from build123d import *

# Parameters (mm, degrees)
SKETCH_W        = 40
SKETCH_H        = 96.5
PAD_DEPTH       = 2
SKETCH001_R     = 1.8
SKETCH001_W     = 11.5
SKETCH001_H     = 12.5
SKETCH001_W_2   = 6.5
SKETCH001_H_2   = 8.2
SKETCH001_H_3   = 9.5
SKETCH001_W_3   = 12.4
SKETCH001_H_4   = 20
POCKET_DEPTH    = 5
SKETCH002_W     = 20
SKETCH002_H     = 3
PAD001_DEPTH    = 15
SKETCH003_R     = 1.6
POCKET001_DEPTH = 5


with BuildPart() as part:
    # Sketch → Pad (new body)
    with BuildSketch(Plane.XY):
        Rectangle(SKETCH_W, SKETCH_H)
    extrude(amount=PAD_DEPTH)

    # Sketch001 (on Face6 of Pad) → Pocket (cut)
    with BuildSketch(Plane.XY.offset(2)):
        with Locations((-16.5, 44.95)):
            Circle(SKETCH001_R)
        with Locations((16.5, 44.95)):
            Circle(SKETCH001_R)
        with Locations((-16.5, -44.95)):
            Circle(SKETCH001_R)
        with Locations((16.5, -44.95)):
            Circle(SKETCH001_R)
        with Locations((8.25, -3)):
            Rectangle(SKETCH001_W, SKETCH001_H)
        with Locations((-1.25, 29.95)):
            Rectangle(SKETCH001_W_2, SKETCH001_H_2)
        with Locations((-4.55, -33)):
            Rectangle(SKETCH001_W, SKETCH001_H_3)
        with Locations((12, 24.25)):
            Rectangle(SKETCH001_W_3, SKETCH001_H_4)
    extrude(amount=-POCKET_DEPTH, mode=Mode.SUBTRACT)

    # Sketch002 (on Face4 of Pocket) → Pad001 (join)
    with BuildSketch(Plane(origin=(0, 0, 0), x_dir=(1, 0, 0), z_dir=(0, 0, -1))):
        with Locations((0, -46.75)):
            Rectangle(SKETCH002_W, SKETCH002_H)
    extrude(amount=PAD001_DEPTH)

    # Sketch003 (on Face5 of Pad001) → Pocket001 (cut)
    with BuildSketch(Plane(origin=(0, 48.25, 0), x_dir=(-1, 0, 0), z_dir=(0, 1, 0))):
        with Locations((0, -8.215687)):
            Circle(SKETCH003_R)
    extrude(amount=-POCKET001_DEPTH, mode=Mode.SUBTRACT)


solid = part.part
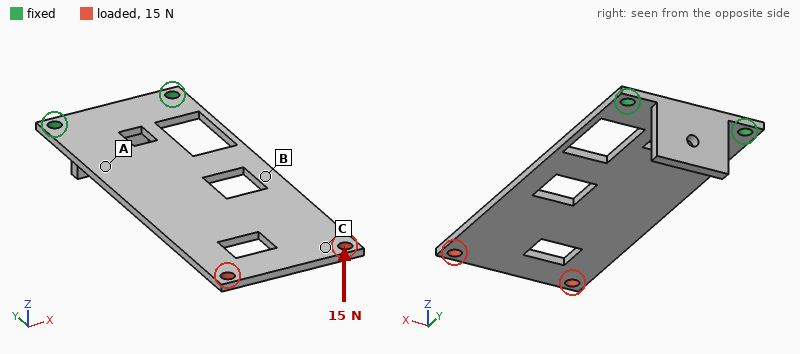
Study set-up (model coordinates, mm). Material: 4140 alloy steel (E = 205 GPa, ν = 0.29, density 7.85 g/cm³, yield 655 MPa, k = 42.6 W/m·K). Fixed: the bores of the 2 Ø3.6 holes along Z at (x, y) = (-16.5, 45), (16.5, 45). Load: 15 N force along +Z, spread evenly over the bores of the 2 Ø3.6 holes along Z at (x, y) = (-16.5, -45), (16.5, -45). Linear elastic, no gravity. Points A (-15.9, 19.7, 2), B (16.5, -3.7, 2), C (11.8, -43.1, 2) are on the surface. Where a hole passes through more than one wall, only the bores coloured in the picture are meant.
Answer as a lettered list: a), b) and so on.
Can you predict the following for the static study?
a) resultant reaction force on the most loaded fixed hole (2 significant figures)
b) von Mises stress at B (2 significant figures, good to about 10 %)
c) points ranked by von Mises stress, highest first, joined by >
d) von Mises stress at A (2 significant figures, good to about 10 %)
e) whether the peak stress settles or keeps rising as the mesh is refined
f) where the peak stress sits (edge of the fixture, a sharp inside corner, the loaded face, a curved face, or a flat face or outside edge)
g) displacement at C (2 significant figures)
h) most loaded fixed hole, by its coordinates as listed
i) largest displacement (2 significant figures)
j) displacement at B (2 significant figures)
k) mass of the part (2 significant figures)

a) 12 N
b) 33 MPa
c) A > B > C
d) 55 MPa
e) keeps rising
f) edge of the fixture
g) 0.99 mm
h) (-16.5, 45)
i) 1.1 mm
j) 0.38 mm
k) 58 g
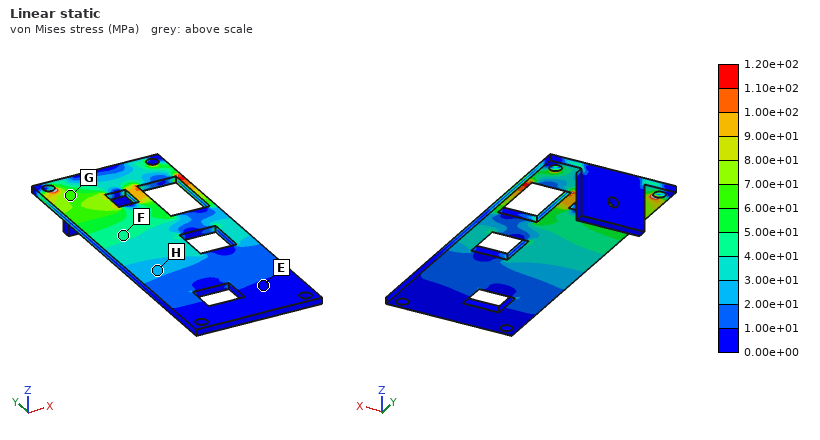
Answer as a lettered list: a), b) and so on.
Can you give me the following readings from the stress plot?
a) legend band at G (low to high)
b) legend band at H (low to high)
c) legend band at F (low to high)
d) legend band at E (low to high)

a) 6.00e+01 to 7.00e+01 MPa
b) 2.00e+01 to 3.00e+01 MPa
c) 4.00e+01 to 5.00e+01 MPa
d) 0.00e+00 to 1.00e+01 MPa
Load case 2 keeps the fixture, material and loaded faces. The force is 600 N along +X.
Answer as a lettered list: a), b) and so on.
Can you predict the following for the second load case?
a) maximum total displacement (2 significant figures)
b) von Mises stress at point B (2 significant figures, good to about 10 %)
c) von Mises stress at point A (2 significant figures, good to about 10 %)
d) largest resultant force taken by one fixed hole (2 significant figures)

a) 0.16 mm
b) 68 MPa
c) 65 MPa
d) 1.7 kN
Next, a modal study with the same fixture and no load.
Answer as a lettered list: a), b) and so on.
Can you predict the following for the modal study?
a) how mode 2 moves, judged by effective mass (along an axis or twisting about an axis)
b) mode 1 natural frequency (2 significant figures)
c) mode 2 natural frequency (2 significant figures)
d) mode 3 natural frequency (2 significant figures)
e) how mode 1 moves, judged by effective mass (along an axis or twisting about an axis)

a) twisting about Y
b) 160 Hz
c) 840 Hz
d) 1100 Hz
e) along Z
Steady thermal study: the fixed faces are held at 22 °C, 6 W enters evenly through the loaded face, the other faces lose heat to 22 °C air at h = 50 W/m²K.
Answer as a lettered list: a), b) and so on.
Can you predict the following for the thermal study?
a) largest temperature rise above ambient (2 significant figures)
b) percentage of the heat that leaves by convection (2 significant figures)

a) 68 K
b) 96 %
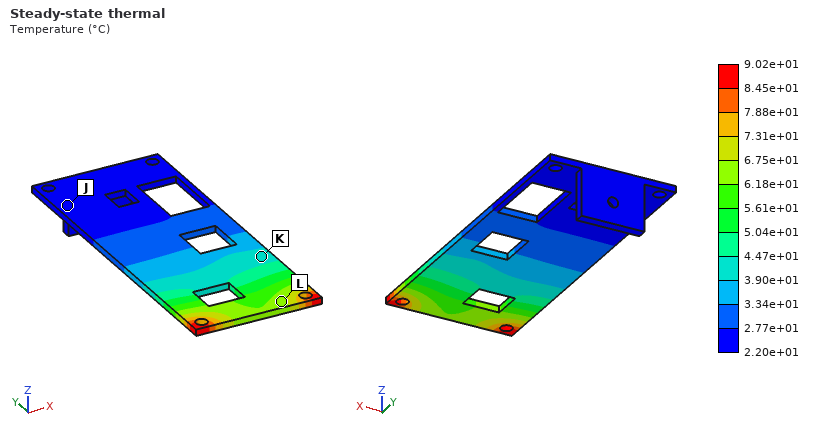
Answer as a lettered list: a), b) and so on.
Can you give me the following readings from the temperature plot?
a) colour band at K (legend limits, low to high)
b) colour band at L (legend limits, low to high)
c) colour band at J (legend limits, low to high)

a) 3.90e+01 to 4.47e+01 °C
b) 6.18e+01 to 6.75e+01 °C
c) 2.20e+01 to 2.77e+01 °C
